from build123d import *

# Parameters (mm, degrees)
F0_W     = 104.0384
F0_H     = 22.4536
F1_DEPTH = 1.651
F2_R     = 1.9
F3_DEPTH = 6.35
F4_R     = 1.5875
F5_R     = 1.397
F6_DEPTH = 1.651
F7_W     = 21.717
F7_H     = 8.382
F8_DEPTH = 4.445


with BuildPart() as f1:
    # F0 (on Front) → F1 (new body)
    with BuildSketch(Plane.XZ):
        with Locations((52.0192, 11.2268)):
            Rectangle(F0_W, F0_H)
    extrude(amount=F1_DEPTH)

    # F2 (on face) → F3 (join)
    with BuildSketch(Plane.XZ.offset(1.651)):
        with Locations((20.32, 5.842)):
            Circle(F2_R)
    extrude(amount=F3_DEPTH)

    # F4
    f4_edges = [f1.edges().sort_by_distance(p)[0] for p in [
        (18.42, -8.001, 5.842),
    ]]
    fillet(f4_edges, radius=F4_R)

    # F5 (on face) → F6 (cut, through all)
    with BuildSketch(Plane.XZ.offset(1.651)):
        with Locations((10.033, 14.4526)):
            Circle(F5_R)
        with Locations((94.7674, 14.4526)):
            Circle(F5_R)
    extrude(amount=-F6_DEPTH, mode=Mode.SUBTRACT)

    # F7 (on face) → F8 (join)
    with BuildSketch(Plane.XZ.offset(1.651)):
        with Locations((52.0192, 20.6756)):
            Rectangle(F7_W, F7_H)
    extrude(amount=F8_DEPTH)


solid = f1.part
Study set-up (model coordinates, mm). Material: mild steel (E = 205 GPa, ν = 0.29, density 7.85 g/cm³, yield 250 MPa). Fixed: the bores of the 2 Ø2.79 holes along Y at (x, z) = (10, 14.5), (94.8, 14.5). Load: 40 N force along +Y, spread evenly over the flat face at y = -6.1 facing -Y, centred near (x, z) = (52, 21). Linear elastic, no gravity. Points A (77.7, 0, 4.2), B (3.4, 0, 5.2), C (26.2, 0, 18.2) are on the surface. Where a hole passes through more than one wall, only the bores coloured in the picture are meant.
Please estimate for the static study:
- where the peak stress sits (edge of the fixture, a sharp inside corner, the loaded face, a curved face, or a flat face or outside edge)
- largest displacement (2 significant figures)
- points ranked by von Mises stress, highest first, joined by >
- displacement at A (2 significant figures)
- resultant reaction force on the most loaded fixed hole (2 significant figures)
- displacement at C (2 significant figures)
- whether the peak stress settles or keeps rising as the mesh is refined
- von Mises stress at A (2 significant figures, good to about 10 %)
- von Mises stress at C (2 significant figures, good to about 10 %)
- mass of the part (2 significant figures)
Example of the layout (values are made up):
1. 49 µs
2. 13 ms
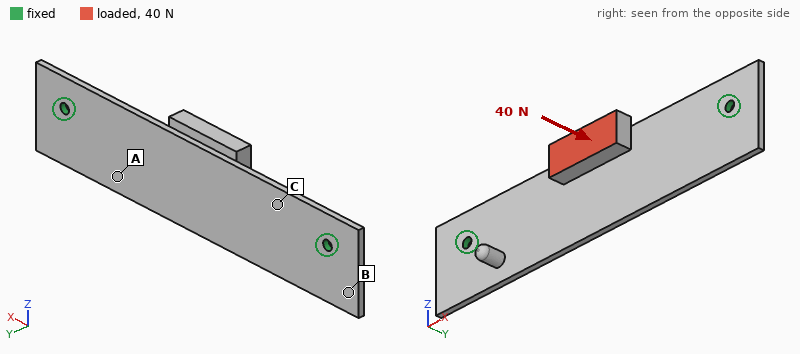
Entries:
1. edge of the fixture
2. 64 µm
3. C > A > B
4. 13 µm
5. 29 N
6. 25 µm
7. keeps rising
8. 10 MPa
9. 18 MPa
10. 37 g
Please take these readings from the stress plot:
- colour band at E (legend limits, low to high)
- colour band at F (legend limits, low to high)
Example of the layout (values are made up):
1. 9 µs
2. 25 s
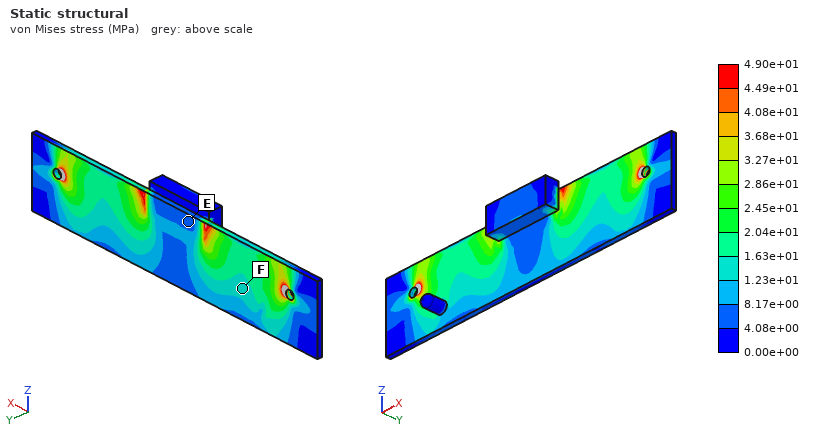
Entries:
1. 4.08e+00 to 8.17e+00 MPa
2. 1.23e+01 to 1.63e+01 MPa
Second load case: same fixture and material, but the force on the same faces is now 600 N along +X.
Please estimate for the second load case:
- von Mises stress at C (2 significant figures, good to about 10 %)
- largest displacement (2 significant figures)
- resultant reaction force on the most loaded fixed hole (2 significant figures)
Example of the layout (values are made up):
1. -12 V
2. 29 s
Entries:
1. 19 MPa
2. 65 µm
3. 310 N
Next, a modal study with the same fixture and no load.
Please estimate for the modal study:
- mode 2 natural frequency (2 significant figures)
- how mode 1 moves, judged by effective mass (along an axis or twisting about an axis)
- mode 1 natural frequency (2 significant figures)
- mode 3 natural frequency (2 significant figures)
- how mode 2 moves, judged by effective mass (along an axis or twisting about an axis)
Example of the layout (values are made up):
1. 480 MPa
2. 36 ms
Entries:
1. 2000 Hz
2. along Y
3. 1100 Hz
4. 3000 Hz
5. twisting about X
